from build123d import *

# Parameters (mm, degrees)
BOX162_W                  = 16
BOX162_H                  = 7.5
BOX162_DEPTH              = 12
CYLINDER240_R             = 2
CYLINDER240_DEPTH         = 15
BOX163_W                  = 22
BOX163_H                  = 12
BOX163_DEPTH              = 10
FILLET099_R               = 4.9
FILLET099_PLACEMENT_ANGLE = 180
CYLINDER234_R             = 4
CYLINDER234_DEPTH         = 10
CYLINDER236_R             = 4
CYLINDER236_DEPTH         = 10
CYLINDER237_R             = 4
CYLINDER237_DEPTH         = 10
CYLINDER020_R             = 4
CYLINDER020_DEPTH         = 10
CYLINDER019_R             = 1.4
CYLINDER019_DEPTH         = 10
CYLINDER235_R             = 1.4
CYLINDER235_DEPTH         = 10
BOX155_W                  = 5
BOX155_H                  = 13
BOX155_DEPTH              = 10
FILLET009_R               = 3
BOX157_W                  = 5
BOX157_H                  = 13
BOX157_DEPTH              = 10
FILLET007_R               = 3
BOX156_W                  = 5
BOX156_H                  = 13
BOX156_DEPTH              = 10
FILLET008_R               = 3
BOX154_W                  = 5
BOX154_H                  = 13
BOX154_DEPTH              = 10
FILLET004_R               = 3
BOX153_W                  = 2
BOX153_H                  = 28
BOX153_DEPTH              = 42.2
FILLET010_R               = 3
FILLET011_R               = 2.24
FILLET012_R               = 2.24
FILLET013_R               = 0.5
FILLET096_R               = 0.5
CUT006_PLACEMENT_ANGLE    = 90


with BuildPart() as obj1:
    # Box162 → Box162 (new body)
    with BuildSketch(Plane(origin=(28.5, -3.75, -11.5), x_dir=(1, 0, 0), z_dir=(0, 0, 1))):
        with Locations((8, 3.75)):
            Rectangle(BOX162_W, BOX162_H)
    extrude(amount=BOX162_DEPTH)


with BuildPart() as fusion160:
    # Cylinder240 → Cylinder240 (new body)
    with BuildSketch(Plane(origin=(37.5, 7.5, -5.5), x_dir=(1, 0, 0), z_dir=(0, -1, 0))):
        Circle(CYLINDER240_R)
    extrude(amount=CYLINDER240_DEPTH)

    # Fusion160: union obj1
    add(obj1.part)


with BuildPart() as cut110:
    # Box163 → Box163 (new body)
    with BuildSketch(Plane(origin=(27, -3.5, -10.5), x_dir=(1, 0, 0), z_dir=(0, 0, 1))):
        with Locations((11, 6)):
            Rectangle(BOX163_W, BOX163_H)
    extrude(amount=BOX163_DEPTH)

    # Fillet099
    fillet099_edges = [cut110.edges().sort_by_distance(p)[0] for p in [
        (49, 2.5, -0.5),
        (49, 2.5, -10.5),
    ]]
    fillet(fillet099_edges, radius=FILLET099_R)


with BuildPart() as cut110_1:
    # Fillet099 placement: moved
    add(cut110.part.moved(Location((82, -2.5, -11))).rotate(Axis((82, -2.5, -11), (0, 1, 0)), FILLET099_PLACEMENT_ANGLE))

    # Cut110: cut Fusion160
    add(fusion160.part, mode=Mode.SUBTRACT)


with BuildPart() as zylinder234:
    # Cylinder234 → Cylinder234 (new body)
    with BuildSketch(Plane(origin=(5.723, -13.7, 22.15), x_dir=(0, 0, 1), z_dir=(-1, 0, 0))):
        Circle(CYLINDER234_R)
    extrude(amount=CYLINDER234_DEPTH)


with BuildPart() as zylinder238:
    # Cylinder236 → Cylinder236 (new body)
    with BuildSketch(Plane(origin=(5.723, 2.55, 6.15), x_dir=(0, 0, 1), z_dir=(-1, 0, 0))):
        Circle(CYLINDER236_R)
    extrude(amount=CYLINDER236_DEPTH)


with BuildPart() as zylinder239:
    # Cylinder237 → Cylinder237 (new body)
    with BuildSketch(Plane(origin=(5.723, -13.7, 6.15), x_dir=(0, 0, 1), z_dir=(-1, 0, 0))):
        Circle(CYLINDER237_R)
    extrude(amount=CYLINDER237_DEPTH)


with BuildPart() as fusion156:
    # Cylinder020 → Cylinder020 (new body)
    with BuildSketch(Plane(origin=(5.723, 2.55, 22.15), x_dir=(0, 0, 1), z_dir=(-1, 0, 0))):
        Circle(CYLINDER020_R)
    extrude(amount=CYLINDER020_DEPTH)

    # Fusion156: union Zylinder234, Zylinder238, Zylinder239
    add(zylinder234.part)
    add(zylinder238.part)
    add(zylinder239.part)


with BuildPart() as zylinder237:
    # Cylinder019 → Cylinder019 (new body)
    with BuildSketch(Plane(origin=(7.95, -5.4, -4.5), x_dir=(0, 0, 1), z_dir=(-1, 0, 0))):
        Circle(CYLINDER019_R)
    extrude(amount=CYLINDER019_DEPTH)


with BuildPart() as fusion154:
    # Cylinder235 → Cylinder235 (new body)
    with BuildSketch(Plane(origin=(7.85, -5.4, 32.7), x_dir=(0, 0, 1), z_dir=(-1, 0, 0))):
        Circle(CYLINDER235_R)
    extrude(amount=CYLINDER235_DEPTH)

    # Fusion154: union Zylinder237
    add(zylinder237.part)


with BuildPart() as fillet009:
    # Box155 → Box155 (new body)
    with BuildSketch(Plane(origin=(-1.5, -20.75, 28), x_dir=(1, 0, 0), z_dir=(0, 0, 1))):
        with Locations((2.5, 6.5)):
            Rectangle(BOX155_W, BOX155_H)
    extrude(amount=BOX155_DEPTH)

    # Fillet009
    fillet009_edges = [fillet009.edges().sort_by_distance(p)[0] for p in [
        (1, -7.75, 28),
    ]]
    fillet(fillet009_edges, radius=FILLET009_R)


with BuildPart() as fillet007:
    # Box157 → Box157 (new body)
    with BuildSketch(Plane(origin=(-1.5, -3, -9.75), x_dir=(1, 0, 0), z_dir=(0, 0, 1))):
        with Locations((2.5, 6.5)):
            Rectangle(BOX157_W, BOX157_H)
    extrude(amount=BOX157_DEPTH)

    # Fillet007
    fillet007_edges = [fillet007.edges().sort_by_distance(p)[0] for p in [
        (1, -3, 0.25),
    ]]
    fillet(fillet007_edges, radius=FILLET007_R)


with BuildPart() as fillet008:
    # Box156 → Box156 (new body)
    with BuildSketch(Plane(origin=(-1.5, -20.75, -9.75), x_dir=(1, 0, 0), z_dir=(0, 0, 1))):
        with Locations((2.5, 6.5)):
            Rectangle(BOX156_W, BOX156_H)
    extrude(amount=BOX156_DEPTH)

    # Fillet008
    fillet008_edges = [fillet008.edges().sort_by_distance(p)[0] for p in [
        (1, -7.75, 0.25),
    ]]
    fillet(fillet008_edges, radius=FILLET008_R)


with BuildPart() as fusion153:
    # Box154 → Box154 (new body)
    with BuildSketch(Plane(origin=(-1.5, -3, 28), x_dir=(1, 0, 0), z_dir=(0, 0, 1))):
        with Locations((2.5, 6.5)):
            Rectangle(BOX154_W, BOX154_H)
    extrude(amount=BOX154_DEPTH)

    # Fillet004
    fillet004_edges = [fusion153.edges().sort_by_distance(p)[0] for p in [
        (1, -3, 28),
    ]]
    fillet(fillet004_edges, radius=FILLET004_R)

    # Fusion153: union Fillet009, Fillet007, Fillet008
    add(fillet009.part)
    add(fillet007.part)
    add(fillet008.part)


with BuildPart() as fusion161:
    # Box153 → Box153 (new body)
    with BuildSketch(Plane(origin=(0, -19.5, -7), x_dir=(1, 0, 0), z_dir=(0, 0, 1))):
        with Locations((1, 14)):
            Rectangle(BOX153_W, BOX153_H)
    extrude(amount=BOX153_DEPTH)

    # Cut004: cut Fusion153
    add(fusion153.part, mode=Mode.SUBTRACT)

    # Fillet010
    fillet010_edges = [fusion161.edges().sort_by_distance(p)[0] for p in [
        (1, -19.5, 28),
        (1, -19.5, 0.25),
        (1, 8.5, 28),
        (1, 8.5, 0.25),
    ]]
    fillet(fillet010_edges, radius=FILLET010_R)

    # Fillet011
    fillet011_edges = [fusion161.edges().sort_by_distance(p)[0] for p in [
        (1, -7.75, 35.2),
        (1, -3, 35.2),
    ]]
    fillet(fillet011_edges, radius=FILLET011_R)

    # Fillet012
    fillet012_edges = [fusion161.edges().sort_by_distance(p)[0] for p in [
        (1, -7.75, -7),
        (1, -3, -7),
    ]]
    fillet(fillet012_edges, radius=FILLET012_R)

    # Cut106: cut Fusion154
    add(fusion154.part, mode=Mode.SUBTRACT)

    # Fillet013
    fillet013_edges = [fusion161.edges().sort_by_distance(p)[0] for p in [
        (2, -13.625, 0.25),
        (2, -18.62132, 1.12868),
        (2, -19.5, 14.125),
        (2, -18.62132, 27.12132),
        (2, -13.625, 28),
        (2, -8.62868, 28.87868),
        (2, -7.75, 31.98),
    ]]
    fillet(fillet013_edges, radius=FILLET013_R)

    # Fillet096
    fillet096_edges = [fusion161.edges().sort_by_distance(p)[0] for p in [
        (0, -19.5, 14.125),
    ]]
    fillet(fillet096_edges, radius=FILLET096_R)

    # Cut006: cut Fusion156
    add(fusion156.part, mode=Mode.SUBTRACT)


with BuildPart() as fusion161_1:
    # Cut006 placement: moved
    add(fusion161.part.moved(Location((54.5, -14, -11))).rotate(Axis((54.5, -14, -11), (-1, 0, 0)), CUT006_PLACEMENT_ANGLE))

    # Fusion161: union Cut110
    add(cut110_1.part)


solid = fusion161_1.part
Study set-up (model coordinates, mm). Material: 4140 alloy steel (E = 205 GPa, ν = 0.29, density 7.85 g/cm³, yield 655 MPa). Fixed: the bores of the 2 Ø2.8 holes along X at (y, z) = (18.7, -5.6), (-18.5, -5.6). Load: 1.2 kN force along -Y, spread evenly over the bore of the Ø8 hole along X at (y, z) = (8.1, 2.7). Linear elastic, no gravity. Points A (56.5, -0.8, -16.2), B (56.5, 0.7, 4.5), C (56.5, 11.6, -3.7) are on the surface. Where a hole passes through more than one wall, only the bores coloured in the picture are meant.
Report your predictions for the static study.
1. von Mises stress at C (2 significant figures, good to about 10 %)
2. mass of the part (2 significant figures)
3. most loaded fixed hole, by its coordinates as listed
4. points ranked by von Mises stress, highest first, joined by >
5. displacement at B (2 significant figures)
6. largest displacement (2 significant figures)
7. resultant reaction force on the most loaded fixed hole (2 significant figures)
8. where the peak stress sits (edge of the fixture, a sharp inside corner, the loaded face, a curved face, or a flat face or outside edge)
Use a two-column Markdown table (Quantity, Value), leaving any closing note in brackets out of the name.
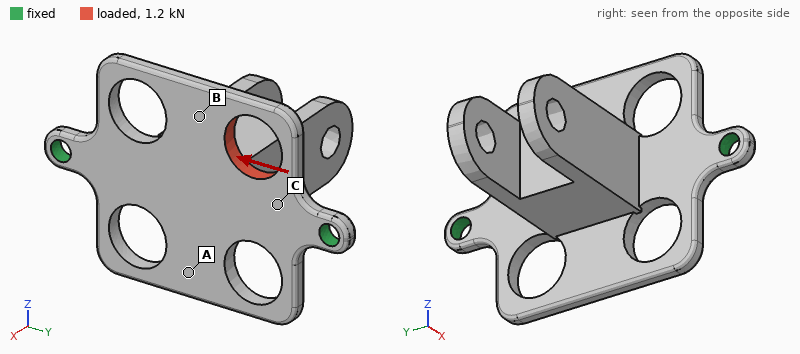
| Quantity | Value |
|---|---|
| von Mises stress at C | 65 MPa |
| mass of the part | 22 g |
| most loaded fixed hole, by its coordinates as listed | (18.7, -5.6) |
| points ranked by von Mises stress, highest first, joined by > | C > B > A |
| displacement at B | 8.7 µm |
| largest displacement | 15 µm |
| resultant reaction force on the most loaded fixed hole | 750 N |
| where the peak stress sits | a curved face |
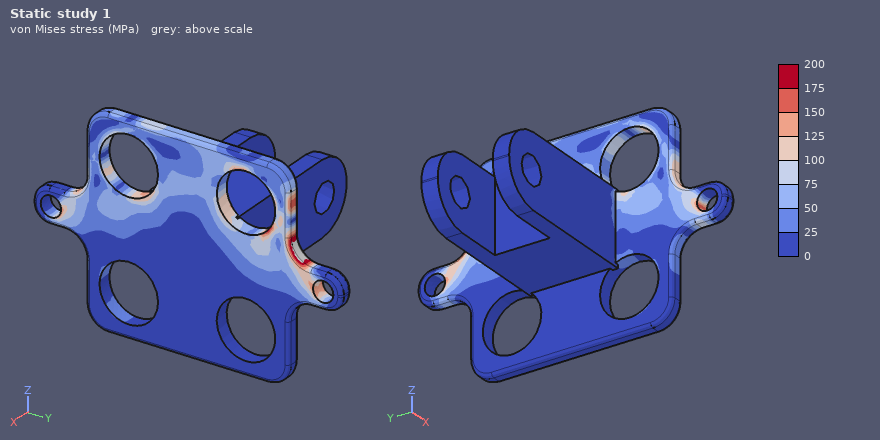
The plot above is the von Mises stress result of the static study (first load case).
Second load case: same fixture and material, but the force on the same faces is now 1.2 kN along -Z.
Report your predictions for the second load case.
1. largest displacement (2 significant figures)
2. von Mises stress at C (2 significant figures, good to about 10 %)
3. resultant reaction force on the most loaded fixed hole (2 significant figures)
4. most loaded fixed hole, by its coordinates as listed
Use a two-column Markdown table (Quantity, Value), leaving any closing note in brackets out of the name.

| Quantity | Value |
|---|---|
| largest displacement | 17 µm |
| von Mises stress at C | 43 MPa |
| resultant reaction force on the most loaded fixed hole | 900 N |
| most loaded fixed hole, by its coordinates as listed | (18.7, -5.6) |
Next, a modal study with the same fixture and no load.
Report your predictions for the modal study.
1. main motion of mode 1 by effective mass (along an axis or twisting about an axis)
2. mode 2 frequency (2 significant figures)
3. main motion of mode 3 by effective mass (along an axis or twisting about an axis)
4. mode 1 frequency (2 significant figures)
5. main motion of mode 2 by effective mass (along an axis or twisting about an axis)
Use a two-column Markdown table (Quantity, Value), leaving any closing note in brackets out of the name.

| Quantity | Value |
|---|---|
| main motion of mode 1 by effective mass | along Z |
| mode 2 frequency | 3800 Hz |
| main motion of mode 3 by effective mass | along Y |
| mode 1 frequency | 1900 Hz |
| main motion of mode 2 by effective mass | along X |
